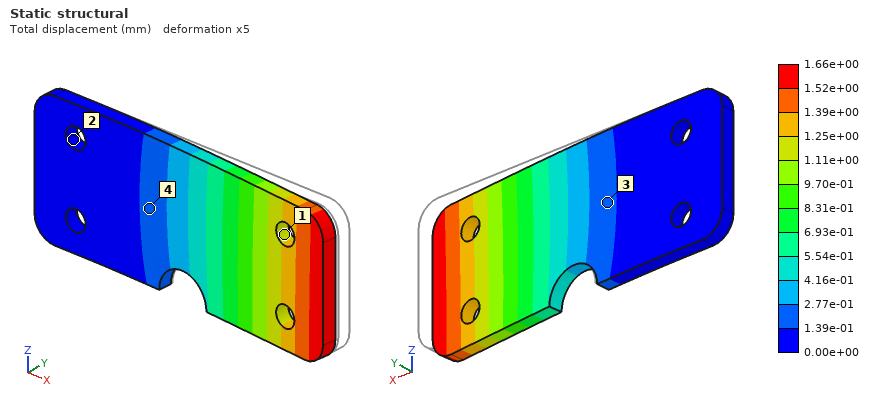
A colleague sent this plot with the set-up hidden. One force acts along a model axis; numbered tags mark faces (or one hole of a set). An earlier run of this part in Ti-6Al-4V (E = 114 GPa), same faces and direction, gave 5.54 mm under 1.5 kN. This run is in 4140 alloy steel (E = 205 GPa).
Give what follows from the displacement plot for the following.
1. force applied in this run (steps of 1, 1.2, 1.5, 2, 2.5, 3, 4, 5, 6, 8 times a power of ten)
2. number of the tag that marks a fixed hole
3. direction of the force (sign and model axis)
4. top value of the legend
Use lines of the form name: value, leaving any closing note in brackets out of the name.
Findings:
force applied in this run: 800 N
number of the tag that marks a fixed hole: 2
direction of the force: -Y
top value of the legend: 1.66e+00 mm
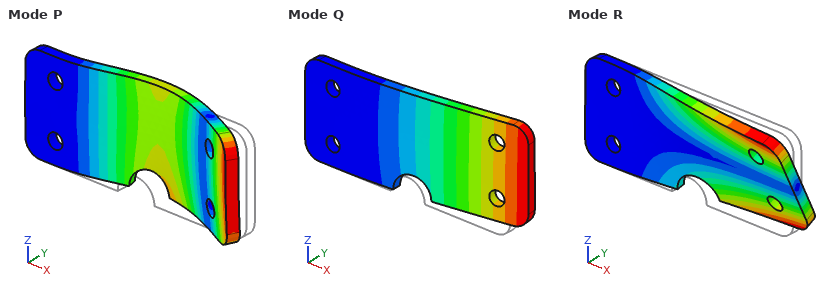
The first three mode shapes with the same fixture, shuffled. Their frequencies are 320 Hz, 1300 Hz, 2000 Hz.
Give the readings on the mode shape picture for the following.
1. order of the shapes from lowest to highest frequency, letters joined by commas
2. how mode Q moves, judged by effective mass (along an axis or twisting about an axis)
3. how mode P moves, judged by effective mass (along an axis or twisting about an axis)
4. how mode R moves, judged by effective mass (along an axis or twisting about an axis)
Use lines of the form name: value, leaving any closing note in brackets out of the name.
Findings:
order of the shapes from lowest to highest frequency, letters joined by commas: Q, R, P
how mode Q moves, judged by effective mass: along Y
how mode P moves, judged by effective mass: along Y
how mode R moves, judged by effective mass: twisting about X
